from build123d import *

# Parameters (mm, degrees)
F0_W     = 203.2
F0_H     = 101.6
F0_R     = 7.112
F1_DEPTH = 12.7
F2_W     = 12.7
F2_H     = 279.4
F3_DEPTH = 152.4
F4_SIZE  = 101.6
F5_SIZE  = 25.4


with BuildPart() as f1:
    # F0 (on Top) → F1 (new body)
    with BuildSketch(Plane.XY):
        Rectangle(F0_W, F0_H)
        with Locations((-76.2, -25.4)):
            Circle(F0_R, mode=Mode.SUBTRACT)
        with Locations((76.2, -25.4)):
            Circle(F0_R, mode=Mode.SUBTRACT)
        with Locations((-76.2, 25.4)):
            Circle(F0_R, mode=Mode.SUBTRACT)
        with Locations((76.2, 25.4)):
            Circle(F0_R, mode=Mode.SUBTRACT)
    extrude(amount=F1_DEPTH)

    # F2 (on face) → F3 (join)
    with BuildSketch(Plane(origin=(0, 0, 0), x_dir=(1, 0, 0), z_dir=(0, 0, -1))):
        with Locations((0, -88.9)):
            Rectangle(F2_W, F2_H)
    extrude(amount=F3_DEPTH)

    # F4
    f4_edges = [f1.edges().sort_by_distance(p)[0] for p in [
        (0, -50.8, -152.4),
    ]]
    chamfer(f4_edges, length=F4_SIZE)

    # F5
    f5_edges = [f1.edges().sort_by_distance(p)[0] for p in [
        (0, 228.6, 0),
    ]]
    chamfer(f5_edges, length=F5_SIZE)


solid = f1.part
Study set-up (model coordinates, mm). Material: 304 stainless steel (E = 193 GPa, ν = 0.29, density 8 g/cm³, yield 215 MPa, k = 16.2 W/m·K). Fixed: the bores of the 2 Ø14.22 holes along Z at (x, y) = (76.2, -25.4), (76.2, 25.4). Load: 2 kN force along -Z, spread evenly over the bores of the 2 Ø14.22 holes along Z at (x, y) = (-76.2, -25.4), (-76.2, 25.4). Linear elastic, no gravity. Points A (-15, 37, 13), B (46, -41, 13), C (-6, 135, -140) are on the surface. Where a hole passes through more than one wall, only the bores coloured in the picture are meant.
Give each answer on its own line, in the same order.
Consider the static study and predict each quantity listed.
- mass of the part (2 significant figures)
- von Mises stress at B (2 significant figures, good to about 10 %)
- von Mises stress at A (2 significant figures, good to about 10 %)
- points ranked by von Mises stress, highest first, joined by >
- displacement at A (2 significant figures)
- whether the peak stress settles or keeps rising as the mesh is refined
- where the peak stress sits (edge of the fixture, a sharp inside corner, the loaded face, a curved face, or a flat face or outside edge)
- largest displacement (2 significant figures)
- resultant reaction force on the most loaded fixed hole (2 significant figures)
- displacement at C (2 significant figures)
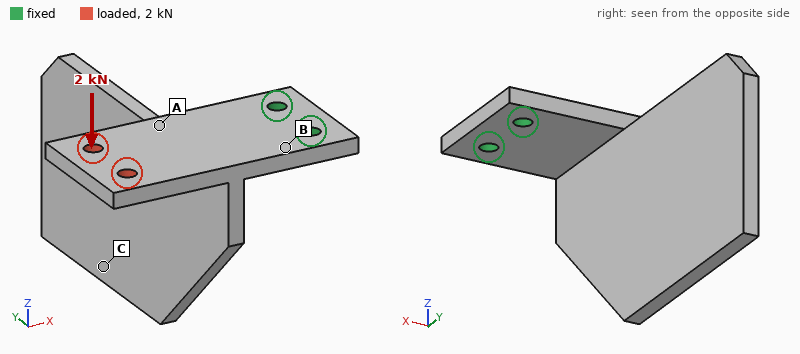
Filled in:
5.8 kg
87 MPa
40 MPa
B > A > C
0.27 mm
keeps rising
edge of the fixture
0.80 mm
1.0 kN
0.73 mm
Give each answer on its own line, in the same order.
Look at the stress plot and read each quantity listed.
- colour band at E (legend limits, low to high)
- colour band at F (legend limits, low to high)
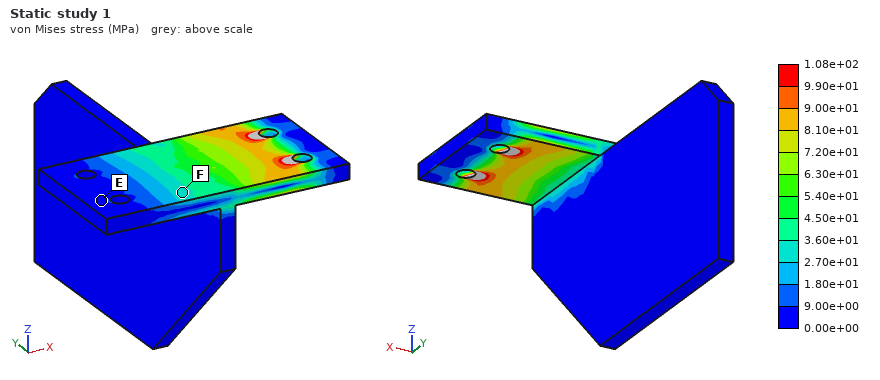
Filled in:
0.00e+00 to 9.00e+00 MPa
2.70e+01 to 3.60e+01 MPa
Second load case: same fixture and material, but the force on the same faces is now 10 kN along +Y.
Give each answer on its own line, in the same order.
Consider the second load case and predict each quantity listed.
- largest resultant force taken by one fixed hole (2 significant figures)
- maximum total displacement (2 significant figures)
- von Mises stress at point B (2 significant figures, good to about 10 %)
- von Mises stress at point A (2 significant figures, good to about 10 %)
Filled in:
26 kN
0.13 mm
42 MPa
23 MPa
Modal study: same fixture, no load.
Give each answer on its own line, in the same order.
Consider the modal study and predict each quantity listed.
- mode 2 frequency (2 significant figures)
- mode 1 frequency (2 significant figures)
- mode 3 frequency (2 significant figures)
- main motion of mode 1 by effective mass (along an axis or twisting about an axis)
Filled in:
190 Hz
120 Hz
280 Hz
along X
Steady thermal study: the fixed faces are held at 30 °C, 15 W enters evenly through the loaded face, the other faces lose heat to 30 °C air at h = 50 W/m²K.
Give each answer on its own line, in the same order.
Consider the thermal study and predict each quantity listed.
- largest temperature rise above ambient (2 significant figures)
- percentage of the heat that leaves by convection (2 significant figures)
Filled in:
22 K
97 %
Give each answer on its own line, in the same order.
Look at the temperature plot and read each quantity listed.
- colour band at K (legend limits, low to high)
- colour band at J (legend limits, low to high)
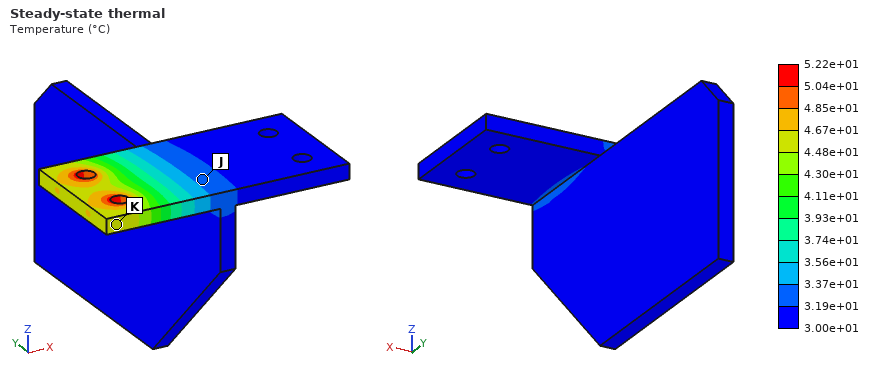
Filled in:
4.48e+01 to 4.67e+01 °C
3.19e+01 to 3.37e+01 °C
